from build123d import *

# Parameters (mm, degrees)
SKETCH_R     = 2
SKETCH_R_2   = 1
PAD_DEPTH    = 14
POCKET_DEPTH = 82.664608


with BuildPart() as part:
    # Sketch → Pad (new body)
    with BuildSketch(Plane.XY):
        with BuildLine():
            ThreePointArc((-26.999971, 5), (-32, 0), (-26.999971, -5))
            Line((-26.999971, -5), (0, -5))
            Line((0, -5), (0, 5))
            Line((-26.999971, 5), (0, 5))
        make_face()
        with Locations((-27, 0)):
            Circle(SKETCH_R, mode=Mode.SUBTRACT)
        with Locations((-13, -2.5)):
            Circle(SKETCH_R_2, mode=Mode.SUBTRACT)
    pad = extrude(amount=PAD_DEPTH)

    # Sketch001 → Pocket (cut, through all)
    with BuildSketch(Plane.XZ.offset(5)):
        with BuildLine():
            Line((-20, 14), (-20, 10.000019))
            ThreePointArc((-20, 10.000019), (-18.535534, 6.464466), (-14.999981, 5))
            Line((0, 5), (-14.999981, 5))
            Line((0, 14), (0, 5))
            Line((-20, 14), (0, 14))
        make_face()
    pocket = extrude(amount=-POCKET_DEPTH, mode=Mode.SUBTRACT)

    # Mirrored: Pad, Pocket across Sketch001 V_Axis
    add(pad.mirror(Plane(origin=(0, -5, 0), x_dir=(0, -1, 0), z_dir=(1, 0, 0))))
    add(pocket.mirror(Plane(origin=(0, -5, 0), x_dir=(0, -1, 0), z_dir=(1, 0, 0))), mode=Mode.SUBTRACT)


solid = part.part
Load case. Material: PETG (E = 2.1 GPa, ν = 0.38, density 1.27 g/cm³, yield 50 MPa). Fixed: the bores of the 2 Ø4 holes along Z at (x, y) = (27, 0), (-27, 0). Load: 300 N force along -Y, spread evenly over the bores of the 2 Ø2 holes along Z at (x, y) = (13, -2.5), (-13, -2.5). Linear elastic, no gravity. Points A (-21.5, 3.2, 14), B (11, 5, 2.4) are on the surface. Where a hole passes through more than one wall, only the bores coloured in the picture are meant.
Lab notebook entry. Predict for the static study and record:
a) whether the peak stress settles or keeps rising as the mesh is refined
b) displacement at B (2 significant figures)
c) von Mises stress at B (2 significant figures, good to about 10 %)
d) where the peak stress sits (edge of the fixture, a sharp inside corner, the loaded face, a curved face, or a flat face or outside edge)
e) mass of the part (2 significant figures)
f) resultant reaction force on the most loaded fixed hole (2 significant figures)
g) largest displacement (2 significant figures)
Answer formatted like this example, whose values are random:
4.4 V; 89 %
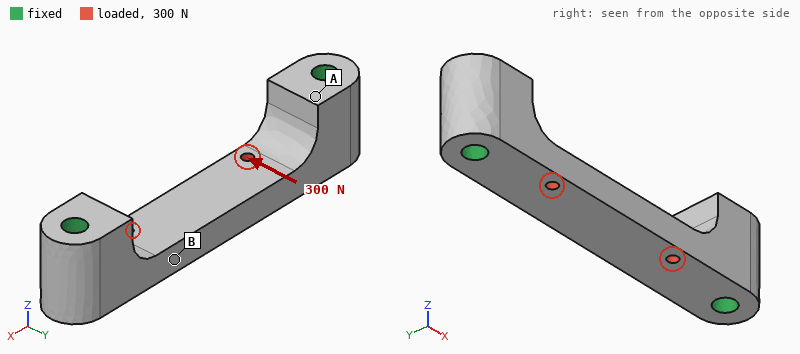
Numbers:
keeps rising; 0.14 mm; 6.5 MPa; edge of the fixture; 6.1 g; 150 N; 0.18 mm
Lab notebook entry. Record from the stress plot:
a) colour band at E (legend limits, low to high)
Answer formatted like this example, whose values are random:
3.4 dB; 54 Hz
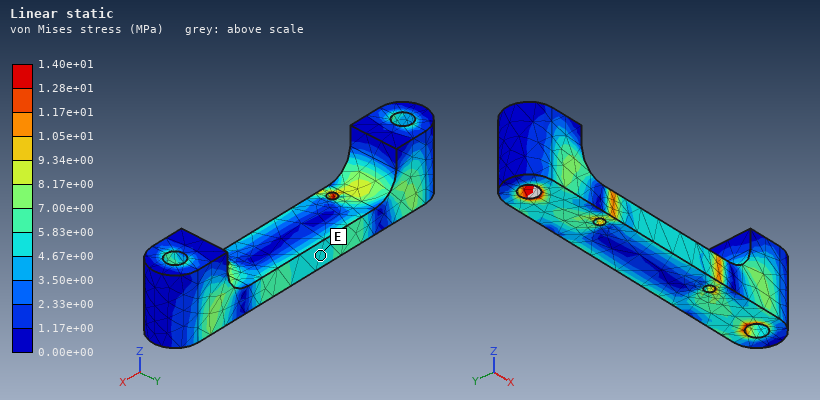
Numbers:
4.67e+00 to 5.83e+00 MPa
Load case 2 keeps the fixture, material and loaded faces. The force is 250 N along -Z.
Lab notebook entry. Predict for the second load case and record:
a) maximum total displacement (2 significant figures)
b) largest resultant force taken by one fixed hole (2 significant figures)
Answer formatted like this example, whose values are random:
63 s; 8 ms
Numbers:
0.20 mm; 130 N
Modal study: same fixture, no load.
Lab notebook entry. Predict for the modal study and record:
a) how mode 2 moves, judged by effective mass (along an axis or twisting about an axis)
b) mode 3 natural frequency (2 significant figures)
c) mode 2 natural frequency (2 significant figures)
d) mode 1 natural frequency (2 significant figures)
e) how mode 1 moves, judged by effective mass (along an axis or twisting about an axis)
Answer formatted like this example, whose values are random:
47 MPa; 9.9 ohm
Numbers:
along Y; 7300 Hz; 4100 Hz; 3600 Hz; along Z
